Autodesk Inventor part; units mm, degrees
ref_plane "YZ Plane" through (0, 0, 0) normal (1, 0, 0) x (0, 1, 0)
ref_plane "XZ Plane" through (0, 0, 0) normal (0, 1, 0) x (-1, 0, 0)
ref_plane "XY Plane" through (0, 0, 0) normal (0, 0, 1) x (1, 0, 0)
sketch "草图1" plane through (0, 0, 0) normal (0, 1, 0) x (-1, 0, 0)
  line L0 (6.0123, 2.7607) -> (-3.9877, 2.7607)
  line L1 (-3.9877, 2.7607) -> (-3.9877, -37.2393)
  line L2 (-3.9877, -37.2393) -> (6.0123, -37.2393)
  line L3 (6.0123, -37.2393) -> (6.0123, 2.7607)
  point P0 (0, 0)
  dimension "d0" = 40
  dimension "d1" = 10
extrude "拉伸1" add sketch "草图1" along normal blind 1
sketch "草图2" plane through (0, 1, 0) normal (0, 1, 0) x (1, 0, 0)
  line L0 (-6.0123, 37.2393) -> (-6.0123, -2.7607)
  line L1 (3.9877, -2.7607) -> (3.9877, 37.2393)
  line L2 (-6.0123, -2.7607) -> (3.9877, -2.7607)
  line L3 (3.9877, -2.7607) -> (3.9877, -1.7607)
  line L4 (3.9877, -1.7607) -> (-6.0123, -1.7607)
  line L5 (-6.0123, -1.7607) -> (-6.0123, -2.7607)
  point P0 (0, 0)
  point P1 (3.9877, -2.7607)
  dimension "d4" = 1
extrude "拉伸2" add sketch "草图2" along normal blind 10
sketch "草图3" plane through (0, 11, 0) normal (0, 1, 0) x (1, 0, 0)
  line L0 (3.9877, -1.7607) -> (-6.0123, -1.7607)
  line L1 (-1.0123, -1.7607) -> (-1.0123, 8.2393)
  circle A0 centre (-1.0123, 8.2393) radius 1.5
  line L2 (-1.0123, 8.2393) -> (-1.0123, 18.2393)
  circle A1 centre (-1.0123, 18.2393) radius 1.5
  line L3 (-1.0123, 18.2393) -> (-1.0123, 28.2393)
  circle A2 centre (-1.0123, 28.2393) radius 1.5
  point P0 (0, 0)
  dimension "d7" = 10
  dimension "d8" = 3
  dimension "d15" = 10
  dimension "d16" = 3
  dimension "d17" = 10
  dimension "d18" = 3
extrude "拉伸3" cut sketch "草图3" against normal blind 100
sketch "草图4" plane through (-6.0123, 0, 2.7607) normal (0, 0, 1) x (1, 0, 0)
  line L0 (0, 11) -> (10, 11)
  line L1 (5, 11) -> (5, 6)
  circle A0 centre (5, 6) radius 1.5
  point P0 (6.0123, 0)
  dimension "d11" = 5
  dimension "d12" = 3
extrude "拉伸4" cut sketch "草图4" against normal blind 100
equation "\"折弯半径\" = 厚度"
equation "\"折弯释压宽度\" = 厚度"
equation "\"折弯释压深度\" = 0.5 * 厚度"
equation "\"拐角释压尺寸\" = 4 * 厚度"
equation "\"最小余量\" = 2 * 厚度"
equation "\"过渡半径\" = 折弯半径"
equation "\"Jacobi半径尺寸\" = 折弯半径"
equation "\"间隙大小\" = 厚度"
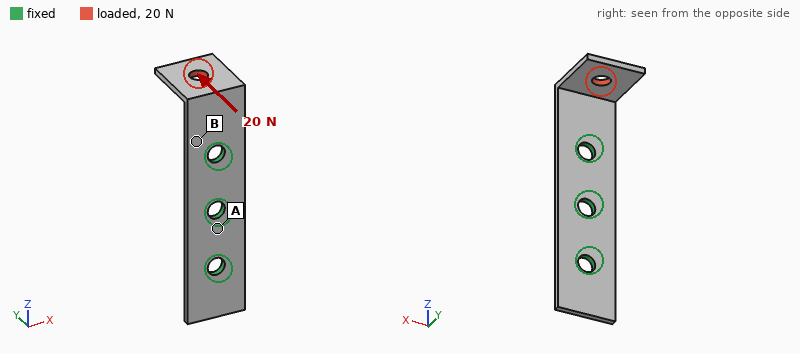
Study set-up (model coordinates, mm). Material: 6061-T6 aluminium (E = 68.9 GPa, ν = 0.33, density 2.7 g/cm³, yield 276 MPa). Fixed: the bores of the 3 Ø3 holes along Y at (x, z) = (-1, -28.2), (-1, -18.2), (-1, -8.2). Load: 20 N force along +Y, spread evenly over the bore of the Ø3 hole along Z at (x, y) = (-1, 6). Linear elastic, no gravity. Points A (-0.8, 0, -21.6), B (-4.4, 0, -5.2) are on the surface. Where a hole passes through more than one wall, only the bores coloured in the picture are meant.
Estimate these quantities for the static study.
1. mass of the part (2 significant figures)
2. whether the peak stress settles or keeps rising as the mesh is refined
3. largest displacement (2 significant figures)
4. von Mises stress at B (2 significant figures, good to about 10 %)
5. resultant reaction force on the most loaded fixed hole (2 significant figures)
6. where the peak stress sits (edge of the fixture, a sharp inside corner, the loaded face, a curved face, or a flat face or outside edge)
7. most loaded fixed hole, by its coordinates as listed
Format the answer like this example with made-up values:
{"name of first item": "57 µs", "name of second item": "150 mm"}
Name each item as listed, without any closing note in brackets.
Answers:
{"mass of the part": "1.3 g", "whether the peak stress settles or keeps rising as the mesh is refined": "keeps rising", "largest displacement": "0.19 mm", "von Mises stress at B": "76 MPa", "resultant reaction force on the most loaded fixed hole": "21 N", "where the peak stress sits": "edge of the fixture", "most loaded fixed hole, by its coordinates as listed": "(-1, -8.2)"}
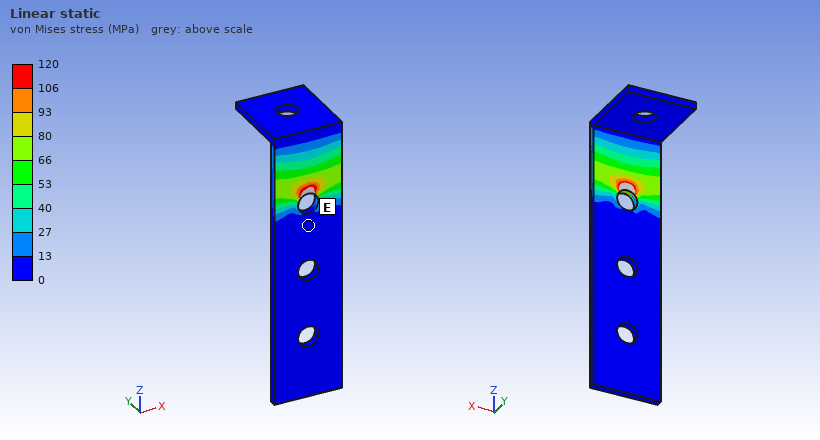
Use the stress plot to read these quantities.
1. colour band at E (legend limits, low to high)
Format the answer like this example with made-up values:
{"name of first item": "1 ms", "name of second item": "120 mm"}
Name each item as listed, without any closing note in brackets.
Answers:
{"colour band at E": "0 to 13 MPa"}
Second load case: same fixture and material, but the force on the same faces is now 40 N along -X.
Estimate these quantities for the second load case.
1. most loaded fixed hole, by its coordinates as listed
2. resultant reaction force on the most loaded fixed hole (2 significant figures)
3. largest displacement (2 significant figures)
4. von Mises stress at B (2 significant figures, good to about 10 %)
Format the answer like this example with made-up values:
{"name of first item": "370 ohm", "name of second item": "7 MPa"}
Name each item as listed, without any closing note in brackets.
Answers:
{"most loaded fixed hole, by its coordinates as listed": "(-1, -8.2)", "resultant reaction force on the most loaded fixed hole": "60 N", "largest displacement": "0.25 mm", "von Mises stress at B": "79 MPa"}
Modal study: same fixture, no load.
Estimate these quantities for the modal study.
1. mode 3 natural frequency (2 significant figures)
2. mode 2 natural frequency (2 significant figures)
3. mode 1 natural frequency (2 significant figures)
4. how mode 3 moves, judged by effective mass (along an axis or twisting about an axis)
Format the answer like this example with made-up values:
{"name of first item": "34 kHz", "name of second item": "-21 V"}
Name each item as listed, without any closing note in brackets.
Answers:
{"mode 3 natural frequency": "7600 Hz", "mode 2 natural frequency": "4500 Hz", "mode 1 natural frequency": "2800 Hz", "how mode 3 moves, judged by effective mass": "along Y"}
